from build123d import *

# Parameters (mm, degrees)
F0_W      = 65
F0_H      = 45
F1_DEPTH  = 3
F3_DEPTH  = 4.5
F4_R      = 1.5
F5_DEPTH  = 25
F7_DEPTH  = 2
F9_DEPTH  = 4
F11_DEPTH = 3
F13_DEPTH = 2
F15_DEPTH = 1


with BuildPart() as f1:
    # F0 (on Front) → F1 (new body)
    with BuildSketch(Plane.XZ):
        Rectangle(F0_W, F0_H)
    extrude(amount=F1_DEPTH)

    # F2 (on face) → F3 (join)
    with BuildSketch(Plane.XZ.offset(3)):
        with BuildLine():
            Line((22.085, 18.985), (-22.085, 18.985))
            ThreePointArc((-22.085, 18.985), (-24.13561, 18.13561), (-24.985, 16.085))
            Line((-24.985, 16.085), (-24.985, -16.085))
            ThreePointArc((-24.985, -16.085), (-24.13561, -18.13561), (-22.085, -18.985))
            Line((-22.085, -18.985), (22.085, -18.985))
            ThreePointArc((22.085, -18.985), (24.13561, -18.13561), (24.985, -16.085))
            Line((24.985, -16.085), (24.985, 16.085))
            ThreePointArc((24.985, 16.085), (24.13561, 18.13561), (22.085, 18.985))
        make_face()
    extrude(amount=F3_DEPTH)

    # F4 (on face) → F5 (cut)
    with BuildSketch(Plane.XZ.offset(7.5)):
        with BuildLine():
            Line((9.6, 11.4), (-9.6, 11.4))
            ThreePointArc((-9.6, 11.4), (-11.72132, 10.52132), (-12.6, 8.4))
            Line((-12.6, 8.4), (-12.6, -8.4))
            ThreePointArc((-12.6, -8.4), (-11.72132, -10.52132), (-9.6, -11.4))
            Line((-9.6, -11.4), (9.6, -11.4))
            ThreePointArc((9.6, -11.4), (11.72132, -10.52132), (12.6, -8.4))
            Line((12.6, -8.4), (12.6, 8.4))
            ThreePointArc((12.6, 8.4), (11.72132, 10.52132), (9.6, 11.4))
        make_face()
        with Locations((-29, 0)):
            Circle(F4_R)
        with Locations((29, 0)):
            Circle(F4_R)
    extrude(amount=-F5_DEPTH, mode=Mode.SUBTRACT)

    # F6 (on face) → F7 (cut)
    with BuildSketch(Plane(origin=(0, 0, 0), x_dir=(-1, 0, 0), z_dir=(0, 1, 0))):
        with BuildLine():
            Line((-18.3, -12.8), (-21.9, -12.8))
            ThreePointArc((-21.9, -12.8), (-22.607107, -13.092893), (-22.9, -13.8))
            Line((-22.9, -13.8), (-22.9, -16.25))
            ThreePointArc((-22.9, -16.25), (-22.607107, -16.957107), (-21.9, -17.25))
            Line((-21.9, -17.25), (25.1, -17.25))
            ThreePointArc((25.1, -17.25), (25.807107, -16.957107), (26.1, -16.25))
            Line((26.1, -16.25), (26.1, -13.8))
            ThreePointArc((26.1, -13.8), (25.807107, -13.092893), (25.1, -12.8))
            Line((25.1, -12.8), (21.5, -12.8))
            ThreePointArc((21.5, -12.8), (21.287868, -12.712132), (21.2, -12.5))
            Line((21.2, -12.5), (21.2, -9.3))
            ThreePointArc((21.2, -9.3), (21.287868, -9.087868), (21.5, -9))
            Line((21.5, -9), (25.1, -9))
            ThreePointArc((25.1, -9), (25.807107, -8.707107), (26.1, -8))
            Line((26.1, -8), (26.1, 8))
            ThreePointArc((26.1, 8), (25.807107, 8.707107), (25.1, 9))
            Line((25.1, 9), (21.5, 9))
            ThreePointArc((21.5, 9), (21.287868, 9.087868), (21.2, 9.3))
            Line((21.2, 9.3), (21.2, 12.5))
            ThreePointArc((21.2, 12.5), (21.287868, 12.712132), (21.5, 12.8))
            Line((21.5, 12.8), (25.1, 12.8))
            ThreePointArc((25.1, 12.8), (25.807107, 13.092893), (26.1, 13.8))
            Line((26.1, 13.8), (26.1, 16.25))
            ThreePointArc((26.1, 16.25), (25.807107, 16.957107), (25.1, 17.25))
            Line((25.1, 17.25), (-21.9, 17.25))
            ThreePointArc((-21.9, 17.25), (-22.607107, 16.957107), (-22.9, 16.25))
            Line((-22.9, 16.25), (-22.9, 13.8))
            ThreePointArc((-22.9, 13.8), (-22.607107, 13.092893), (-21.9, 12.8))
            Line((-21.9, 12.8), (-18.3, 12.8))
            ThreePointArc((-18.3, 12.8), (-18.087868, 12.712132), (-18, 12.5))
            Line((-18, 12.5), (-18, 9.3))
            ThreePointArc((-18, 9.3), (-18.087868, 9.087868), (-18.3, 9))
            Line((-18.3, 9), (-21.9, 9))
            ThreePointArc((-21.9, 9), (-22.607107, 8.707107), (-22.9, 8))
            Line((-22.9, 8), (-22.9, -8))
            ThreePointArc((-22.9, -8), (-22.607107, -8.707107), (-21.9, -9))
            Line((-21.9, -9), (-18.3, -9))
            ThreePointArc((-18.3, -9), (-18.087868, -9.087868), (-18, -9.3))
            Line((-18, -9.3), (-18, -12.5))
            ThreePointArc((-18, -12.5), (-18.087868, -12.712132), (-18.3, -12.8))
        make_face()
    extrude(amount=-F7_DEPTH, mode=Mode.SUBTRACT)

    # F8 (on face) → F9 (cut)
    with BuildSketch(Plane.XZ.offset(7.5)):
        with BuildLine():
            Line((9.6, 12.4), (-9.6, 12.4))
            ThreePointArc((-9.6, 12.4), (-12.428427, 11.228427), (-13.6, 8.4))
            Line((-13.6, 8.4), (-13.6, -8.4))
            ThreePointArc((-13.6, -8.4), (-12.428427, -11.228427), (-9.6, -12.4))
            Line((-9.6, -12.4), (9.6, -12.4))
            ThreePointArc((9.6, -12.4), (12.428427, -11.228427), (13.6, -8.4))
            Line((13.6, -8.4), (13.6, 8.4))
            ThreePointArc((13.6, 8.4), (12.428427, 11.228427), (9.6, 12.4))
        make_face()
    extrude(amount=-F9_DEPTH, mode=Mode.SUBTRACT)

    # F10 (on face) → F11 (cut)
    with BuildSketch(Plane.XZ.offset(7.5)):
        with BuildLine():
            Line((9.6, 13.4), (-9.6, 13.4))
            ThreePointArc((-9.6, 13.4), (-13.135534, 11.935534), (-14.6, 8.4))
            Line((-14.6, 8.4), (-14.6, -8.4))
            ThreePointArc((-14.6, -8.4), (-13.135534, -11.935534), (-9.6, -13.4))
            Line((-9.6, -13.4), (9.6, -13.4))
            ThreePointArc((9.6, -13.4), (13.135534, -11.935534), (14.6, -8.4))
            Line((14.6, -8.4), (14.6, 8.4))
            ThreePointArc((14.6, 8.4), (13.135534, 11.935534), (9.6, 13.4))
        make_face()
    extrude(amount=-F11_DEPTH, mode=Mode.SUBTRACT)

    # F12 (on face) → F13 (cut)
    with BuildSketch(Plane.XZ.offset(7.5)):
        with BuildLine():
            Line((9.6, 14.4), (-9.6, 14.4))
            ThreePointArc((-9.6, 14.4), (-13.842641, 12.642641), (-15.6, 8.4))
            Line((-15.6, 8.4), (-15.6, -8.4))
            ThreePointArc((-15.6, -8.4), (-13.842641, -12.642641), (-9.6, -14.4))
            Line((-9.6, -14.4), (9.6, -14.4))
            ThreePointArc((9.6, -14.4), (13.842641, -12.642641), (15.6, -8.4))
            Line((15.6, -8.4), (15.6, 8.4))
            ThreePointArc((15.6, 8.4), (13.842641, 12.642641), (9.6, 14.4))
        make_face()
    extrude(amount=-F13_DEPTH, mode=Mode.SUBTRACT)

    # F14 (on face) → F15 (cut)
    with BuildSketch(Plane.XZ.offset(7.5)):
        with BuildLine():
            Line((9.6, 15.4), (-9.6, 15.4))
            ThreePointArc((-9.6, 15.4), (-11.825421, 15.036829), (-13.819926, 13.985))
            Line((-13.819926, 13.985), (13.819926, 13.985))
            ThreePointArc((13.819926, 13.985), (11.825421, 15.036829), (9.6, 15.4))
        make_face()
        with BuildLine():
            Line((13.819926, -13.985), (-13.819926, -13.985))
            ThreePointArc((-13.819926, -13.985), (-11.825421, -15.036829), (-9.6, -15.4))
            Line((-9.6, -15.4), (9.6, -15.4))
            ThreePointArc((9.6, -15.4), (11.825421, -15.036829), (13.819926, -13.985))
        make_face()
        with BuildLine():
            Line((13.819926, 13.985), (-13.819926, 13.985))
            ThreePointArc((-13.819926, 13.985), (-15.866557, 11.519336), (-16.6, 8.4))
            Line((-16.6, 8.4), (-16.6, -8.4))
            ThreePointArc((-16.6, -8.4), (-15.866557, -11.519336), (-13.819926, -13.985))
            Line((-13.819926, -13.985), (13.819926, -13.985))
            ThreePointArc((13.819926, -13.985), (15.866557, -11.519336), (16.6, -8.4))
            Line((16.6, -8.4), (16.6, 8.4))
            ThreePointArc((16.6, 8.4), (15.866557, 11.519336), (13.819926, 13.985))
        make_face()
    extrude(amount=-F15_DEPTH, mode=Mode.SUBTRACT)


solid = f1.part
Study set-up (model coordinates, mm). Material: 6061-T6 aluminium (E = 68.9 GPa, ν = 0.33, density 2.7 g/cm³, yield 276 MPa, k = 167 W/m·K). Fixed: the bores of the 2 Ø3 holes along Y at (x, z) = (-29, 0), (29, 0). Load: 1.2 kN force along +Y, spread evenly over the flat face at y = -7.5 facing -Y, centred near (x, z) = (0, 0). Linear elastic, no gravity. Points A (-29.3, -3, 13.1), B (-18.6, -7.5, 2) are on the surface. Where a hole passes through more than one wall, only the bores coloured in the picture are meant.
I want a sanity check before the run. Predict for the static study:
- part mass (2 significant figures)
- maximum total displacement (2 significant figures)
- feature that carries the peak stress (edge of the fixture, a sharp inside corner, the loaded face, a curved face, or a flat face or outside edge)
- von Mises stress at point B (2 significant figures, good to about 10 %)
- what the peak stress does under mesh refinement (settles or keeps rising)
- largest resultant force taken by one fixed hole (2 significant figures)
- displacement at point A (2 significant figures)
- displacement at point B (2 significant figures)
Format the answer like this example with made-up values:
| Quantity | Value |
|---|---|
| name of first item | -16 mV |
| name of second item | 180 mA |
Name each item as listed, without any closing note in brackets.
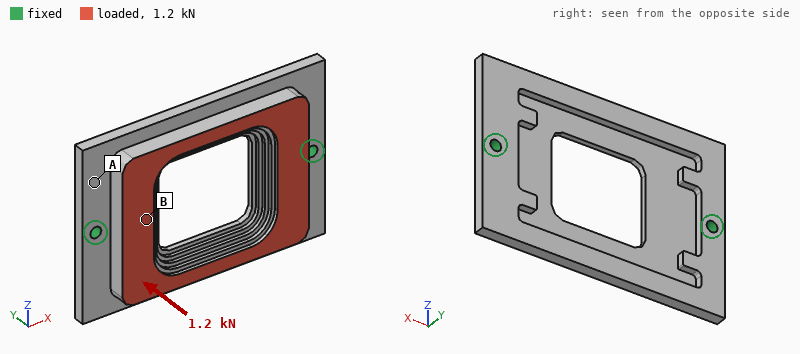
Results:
| Quantity | Value |
|---|---|
| part mass | 27 g |
| maximum total displacement | 79 µm |
| feature that carries the peak stress | edge of the fixture |
| von Mises stress at point B | 35 MPa |
| what the peak stress does under mesh refinement | keeps rising |
| largest resultant force taken by one fixed hole | 880 N |
| displacement at point A | 17 µm |
| displacement at point B | 37 µm |
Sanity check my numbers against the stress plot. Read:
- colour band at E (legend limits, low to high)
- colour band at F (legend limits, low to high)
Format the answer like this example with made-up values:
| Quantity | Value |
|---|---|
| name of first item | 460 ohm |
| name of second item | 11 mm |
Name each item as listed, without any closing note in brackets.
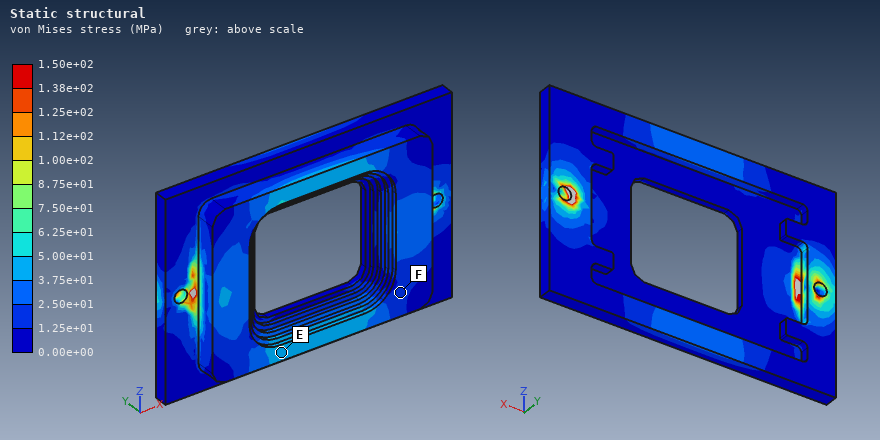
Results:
| Quantity | Value |
|---|---|
| colour band at E | 3.75e+01 to 5.00e+01 MPa |
| colour band at F | 1.25e+01 to 2.50e+01 MPa |
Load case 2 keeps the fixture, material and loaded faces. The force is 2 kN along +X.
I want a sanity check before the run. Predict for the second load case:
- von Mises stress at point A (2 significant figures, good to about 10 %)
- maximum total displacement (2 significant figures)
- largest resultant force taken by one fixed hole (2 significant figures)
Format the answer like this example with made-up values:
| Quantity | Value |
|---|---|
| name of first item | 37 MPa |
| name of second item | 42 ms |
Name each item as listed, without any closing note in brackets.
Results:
| Quantity | Value |
|---|---|
| von Mises stress at point A | 6.1 MPa |
| maximum total displacement | 19 µm |
| largest resultant force taken by one fixed hole | 1.1 kN |
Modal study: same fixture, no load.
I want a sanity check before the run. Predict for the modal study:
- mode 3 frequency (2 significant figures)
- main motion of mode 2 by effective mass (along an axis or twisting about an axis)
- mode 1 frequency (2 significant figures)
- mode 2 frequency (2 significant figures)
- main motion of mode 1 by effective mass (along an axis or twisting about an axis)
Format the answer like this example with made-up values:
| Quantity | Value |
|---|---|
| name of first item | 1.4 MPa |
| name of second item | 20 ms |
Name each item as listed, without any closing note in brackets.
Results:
| Quantity | Value |
|---|---|
| mode 3 frequency | 5700 Hz |
| main motion of mode 2 by effective mass | along Y |
| mode 1 frequency | 2600 Hz |
| mode 2 frequency | 4800 Hz |
| main motion of mode 1 by effective mass | twisting about X |
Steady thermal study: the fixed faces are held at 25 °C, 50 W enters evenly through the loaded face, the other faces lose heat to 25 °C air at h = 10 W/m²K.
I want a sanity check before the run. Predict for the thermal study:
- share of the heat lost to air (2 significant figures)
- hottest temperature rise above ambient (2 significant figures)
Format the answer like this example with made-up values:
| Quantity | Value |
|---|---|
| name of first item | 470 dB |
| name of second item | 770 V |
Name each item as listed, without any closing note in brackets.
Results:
| Quantity | Value |
|---|---|
| share of the heat lost to air | 3.1 % |
| hottest temperature rise above ambient | 32 K |
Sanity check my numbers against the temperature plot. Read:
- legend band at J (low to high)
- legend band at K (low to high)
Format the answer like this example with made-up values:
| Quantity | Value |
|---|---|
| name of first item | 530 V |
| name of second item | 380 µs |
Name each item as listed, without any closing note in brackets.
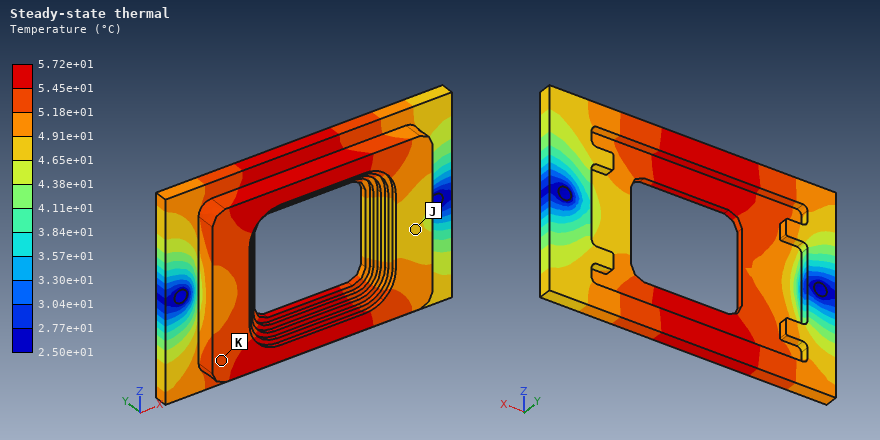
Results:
| Quantity | Value |
|---|---|
| legend band at J | 4.65e+01 to 4.91e+01 °C |
| legend band at K | 5.18e+01 to 5.45e+01 °C |
